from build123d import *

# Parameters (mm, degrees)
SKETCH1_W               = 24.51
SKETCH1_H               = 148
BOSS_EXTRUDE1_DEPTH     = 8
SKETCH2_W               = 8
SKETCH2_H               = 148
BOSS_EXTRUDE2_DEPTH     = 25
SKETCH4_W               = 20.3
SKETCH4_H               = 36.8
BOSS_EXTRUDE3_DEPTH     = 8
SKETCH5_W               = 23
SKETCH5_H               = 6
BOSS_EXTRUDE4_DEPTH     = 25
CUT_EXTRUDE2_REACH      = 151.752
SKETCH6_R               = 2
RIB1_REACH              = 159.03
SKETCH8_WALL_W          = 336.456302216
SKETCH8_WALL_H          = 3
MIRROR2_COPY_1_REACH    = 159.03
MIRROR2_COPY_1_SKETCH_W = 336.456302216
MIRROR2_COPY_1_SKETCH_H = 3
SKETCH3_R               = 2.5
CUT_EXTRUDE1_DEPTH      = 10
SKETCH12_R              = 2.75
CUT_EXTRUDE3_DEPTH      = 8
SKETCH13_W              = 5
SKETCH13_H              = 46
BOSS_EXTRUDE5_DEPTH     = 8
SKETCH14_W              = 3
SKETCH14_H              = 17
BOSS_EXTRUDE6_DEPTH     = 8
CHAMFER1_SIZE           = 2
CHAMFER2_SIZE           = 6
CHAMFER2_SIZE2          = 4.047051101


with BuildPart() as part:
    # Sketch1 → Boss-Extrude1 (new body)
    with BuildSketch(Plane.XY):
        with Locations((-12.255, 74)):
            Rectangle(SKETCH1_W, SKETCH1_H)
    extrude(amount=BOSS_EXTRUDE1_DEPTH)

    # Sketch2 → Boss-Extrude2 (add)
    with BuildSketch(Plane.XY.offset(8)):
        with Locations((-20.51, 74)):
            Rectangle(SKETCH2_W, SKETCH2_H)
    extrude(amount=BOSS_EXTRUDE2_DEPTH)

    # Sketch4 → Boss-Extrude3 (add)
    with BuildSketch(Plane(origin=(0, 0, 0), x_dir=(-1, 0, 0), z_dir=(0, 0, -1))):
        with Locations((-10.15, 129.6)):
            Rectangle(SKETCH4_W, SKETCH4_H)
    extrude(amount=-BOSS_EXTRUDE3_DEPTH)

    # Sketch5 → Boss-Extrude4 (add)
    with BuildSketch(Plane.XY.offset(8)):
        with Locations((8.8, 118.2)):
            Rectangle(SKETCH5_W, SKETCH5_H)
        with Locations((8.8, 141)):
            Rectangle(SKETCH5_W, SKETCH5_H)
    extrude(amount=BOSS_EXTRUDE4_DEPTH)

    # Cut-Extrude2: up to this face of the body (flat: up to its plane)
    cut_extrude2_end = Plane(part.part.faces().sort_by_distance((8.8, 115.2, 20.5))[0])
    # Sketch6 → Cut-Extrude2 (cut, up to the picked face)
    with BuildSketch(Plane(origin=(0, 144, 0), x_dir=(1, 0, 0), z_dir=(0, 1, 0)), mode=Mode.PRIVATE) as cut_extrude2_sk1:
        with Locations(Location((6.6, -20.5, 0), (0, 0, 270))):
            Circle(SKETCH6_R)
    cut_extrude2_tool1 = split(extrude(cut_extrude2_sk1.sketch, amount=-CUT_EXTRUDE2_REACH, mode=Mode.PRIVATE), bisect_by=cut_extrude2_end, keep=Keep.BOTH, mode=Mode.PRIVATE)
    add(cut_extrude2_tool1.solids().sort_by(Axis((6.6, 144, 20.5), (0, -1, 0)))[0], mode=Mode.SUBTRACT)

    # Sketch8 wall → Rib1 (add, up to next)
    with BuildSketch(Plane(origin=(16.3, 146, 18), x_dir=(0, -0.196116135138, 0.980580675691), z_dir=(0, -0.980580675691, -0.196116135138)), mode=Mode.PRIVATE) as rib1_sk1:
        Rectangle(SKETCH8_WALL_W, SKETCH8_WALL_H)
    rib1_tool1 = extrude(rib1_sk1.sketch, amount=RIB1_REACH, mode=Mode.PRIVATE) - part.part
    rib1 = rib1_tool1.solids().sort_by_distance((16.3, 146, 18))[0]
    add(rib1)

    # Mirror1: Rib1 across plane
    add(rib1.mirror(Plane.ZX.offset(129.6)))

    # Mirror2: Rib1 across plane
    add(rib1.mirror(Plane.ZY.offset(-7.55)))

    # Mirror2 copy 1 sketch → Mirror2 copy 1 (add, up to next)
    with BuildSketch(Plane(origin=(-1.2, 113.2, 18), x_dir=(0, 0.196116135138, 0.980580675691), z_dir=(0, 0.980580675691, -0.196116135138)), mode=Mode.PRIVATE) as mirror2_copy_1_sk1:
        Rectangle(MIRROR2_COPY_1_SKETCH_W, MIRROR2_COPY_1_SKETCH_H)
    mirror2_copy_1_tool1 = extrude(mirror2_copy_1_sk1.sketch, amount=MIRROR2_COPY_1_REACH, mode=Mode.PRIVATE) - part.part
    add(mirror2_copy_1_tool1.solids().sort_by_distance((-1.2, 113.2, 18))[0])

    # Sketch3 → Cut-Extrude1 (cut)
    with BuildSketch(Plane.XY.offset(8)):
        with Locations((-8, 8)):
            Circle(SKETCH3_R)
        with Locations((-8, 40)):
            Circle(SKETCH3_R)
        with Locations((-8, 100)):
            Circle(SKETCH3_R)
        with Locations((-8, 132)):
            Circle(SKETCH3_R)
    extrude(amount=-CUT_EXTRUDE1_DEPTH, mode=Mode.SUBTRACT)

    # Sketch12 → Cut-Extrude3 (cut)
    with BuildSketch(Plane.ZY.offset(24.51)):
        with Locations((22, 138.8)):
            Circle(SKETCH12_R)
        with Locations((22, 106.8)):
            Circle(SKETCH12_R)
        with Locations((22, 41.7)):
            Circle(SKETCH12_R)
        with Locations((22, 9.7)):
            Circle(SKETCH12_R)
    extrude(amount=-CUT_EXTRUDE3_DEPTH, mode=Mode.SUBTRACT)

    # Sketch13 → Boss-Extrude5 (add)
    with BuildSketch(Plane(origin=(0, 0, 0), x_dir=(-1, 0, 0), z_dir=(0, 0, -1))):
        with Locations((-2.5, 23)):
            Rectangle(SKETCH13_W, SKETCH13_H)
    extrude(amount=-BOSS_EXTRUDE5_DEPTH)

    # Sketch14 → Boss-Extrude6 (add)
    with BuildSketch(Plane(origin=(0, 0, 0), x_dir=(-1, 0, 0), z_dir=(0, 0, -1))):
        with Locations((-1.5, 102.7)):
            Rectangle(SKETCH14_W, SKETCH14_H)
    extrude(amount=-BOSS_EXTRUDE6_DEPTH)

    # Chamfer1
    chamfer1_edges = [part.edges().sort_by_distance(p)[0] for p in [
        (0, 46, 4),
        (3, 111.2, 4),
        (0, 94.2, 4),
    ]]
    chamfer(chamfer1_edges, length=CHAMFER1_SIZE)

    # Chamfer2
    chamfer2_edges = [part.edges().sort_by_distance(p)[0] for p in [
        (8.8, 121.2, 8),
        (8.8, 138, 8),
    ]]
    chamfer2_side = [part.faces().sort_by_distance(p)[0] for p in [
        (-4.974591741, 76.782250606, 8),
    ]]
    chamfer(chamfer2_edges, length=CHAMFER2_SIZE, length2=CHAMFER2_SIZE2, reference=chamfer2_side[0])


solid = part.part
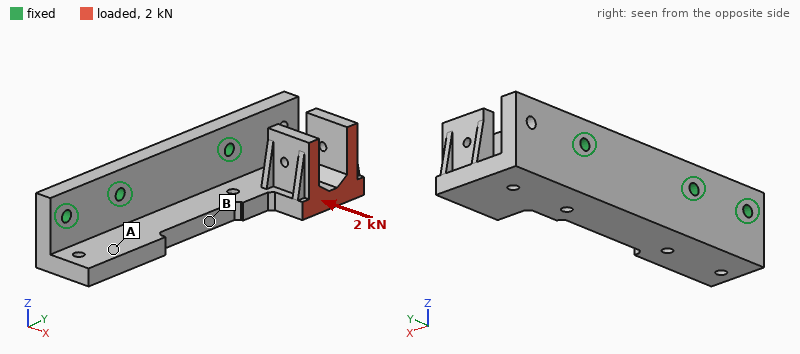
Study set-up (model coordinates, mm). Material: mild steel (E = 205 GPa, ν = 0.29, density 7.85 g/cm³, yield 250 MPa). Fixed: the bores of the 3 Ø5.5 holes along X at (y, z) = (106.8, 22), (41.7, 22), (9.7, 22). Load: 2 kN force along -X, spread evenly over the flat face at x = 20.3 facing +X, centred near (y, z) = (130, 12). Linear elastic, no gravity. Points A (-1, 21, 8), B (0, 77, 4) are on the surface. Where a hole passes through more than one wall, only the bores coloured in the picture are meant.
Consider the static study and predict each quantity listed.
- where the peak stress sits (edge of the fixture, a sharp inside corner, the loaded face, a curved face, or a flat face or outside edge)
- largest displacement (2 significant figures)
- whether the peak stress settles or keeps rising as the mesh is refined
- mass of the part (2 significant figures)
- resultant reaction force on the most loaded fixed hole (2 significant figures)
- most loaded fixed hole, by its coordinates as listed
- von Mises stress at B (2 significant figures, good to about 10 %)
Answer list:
edge of the fixture
51 µm
keeps rising
580 g
2.4 kN
(106.8, 22)
20 MPa
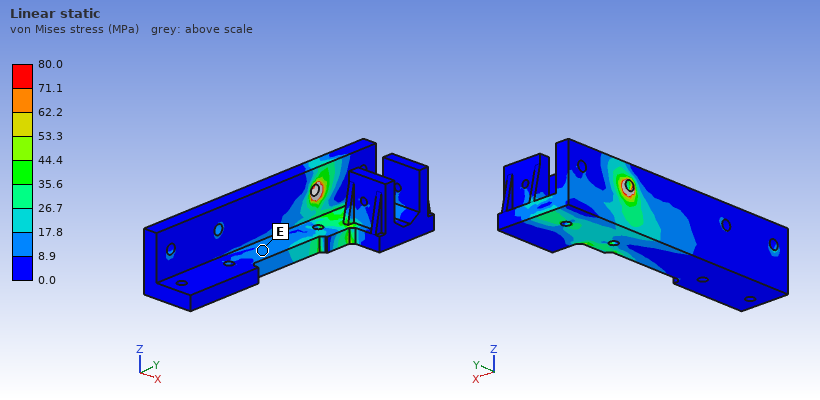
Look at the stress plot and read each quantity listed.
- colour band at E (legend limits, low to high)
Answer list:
8.9 to 17.8 MPa
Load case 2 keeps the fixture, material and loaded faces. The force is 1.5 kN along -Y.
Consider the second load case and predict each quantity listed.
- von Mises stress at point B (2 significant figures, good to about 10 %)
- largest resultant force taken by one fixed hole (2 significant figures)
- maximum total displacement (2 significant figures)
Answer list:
28 MPa
900 N
64 µm
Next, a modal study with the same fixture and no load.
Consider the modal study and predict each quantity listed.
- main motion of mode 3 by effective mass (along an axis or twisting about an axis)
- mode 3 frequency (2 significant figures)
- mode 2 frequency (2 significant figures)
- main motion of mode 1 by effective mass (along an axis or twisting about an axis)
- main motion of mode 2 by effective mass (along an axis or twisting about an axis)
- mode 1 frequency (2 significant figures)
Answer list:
along X
4000 Hz
2800 Hz
along Z
along X
1700 Hz
